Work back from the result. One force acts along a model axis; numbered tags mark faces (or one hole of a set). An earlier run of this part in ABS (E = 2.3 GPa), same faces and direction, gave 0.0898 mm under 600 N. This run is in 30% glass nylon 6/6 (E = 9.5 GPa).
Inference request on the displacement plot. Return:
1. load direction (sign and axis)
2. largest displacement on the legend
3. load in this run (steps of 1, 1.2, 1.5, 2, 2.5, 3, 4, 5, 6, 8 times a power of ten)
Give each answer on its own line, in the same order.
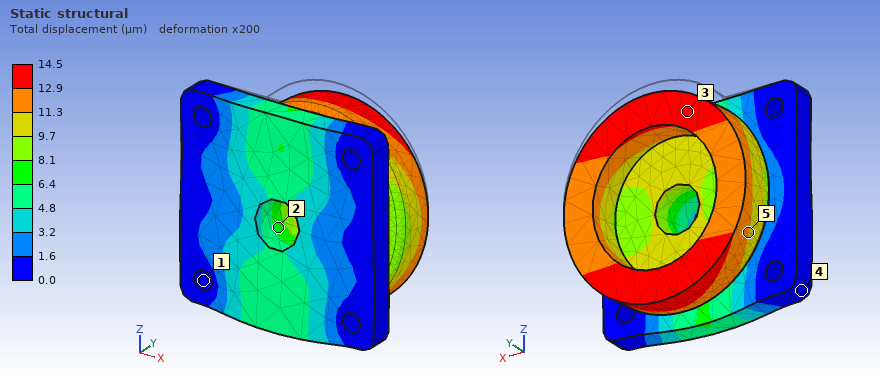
-Z
14.5 µm
400 N
